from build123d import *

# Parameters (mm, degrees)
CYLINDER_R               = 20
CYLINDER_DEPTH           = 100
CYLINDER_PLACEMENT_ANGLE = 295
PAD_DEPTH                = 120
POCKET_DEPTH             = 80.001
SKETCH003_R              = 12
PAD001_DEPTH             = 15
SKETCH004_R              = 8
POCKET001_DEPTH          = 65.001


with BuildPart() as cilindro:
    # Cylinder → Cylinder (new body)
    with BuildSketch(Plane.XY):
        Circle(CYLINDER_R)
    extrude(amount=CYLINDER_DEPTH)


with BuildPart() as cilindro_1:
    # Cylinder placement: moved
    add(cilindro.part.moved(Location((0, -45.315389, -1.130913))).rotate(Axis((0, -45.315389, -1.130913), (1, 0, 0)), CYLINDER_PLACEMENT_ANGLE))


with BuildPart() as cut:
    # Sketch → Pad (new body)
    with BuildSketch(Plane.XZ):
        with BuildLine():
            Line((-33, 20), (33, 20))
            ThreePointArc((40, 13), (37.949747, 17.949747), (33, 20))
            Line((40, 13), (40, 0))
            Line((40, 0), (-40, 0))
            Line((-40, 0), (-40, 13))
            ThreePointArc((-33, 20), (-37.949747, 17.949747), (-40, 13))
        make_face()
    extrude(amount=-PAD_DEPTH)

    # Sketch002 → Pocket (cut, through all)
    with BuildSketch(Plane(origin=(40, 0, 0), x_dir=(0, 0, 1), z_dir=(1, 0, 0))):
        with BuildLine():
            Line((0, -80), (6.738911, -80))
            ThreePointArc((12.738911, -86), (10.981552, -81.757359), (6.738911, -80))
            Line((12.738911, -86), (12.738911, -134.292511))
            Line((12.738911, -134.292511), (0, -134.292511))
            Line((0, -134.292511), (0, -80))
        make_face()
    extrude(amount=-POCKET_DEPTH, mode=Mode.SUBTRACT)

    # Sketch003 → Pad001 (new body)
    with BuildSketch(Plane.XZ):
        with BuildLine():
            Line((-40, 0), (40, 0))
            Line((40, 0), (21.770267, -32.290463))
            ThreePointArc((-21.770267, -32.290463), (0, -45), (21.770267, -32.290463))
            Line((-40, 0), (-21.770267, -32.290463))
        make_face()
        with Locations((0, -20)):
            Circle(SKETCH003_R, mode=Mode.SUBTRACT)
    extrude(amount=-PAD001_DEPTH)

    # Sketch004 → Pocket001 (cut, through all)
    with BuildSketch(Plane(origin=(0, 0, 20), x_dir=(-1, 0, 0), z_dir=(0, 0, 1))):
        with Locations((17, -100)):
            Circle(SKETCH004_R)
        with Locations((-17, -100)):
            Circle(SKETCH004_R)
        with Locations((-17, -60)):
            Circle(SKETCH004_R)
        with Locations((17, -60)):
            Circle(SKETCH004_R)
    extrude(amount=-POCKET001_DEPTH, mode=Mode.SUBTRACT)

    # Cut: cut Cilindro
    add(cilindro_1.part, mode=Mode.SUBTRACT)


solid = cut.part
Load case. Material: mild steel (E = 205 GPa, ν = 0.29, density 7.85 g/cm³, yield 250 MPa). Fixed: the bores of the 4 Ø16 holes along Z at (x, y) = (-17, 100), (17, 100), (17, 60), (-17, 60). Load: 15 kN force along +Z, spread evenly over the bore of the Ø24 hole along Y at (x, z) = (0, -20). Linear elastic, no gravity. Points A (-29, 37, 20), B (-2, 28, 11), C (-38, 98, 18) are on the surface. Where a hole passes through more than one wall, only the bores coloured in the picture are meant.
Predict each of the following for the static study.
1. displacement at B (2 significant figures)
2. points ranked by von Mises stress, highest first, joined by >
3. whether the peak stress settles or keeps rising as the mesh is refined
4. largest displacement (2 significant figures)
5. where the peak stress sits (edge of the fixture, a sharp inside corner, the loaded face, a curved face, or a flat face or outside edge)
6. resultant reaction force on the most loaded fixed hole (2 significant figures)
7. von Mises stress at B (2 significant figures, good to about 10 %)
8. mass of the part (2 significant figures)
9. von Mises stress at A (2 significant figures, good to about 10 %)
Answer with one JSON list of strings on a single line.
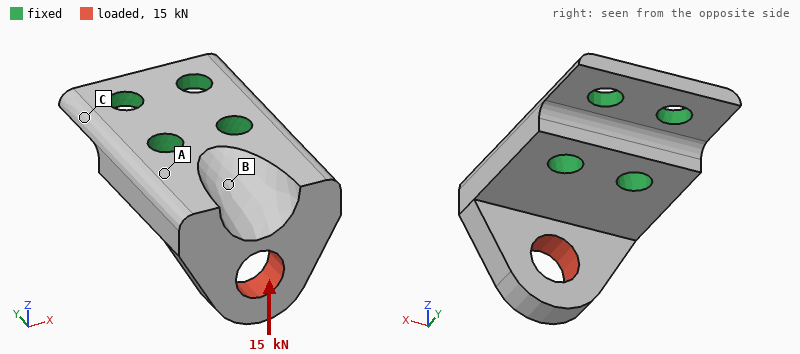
["0.024 mm", "A > B > C", "keeps rising", "0.14 mm", "edge of the fixture", "8.0 kN", "56 MPa", "1.2 kg", "95 MPa"]
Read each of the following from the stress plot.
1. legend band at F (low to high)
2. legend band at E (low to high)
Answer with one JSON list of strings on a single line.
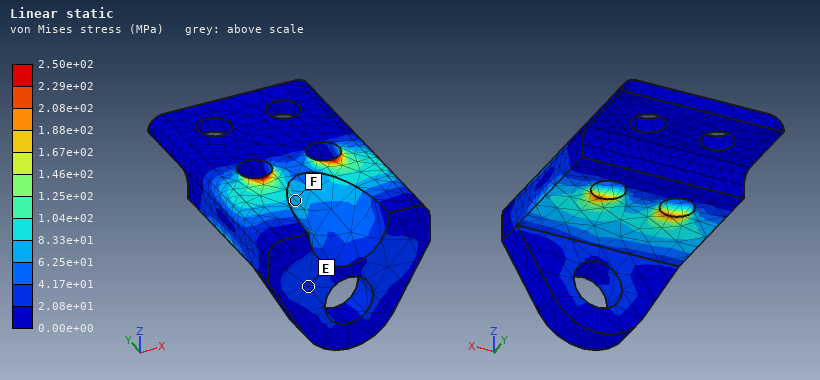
["6.25e+01 to 8.33e+01 MPa", "2.08e+01 to 4.17e+01 MPa"]
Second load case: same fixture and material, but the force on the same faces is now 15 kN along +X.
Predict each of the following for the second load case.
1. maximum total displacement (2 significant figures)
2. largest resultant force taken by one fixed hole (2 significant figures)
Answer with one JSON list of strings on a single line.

["80 µm", "18 kN"]
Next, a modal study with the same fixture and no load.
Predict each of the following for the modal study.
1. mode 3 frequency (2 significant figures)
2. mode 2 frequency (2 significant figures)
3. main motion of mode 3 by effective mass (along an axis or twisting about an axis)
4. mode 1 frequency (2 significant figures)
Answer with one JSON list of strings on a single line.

["6100 Hz", "4400 Hz", "along Z", "2900 Hz"]
